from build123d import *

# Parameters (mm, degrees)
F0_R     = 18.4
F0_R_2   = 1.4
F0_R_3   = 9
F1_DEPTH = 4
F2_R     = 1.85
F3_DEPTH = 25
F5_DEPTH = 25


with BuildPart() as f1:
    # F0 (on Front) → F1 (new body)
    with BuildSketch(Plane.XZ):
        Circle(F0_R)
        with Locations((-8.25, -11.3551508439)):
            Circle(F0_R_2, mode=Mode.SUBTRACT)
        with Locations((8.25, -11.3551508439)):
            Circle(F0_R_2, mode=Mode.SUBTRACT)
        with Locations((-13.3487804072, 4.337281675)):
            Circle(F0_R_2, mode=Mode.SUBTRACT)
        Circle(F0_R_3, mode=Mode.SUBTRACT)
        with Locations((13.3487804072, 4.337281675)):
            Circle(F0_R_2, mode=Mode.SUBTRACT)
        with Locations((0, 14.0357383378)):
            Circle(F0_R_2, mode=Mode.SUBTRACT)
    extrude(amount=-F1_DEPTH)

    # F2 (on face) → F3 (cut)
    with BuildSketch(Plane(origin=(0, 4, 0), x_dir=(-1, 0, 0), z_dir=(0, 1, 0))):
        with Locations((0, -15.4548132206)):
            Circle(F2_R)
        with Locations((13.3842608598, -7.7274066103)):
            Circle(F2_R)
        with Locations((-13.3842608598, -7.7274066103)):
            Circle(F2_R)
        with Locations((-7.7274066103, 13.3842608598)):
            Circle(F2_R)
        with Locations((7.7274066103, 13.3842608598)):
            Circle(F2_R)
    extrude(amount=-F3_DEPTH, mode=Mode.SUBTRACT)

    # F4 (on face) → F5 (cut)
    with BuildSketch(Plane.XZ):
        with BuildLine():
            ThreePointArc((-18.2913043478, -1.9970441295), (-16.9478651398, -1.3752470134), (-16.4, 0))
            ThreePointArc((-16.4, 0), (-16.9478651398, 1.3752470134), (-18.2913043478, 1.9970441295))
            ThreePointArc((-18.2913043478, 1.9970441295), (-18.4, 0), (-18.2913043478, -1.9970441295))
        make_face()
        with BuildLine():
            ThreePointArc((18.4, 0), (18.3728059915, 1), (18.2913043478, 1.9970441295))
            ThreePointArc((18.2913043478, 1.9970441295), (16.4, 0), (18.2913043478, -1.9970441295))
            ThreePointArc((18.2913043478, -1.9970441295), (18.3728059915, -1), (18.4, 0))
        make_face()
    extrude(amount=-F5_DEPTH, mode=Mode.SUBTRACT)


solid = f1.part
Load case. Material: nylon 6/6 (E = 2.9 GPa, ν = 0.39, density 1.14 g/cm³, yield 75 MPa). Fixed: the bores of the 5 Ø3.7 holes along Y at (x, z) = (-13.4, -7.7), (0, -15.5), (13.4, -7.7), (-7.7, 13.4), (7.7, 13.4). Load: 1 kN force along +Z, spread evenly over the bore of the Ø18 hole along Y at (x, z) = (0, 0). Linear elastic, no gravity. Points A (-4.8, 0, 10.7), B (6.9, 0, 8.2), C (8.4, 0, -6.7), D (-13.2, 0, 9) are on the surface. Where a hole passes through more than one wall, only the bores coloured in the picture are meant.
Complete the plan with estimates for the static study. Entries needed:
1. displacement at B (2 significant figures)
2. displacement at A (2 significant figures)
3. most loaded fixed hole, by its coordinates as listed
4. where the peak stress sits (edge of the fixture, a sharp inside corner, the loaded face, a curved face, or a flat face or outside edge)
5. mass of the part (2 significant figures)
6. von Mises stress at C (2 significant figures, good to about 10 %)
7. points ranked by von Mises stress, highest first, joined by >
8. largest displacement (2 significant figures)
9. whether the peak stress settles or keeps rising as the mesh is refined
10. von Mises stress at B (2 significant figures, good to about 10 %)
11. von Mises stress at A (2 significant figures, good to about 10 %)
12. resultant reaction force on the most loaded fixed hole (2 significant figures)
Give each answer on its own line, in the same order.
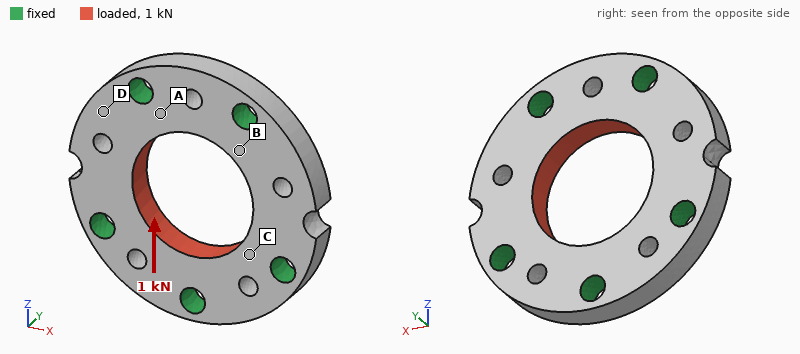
8.1 µm
7.4 µm
(0, -15.5)
edge of the fixture
3.2 g
3.4 MPa
B > A > C > D
21 µm
keeps rising
7.0 MPa
5.5 MPa
250 N
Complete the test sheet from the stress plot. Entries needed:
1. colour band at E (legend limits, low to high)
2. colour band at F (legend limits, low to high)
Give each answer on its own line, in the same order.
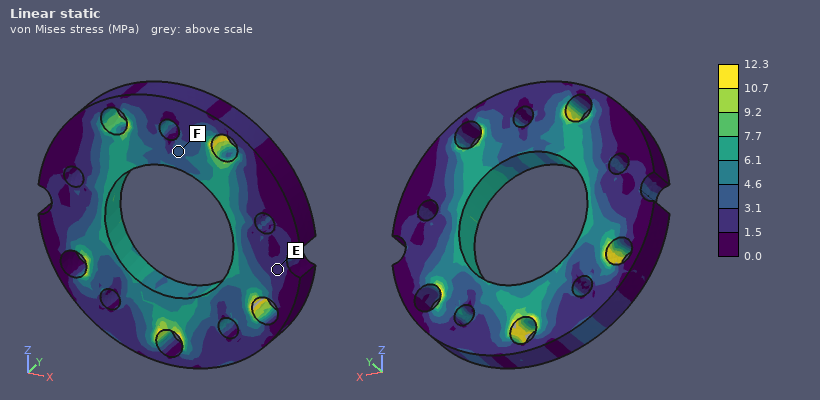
1.5 to 3.1 MPa
3.1 to 4.6 MPa
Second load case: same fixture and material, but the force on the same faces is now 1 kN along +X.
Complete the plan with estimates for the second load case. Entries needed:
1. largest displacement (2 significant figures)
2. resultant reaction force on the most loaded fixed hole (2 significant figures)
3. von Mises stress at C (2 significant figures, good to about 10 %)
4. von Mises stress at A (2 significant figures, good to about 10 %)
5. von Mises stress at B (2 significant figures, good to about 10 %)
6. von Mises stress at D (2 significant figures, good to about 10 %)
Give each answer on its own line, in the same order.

43 µm
230 N
7.9 MPa
7.7 MPa
4.5 MPa
4.0 MPa
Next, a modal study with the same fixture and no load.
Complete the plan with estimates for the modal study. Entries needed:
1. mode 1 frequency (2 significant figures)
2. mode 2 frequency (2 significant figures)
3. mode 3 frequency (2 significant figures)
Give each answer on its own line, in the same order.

11 kHz
11 kHz
18 kHz
